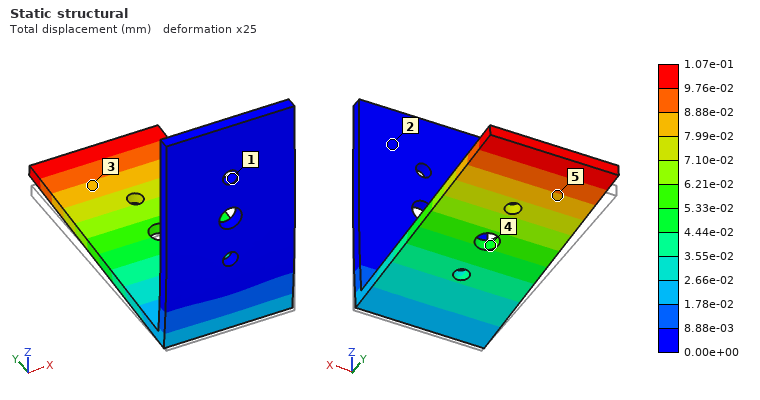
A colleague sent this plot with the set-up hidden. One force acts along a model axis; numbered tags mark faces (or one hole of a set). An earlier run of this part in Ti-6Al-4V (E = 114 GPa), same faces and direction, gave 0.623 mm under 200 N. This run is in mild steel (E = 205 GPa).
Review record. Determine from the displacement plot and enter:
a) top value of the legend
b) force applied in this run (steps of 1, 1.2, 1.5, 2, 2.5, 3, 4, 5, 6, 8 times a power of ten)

1.07e-01 mm
60 N
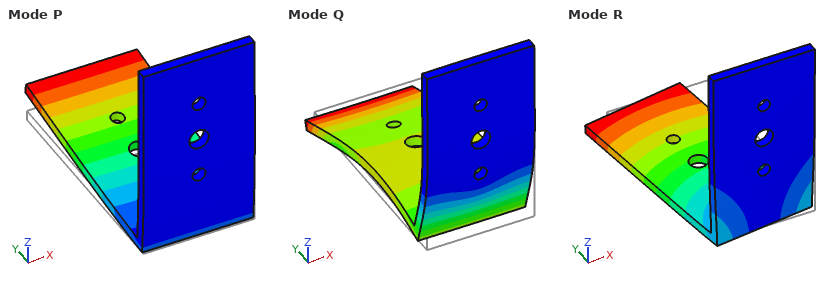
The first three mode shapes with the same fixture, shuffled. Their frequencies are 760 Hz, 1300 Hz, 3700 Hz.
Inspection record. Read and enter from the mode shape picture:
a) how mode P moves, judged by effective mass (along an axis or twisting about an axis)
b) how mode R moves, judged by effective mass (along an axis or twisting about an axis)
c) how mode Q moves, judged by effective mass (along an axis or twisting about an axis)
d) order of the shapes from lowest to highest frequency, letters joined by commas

along Z
along X
along Y
P, R, Q
